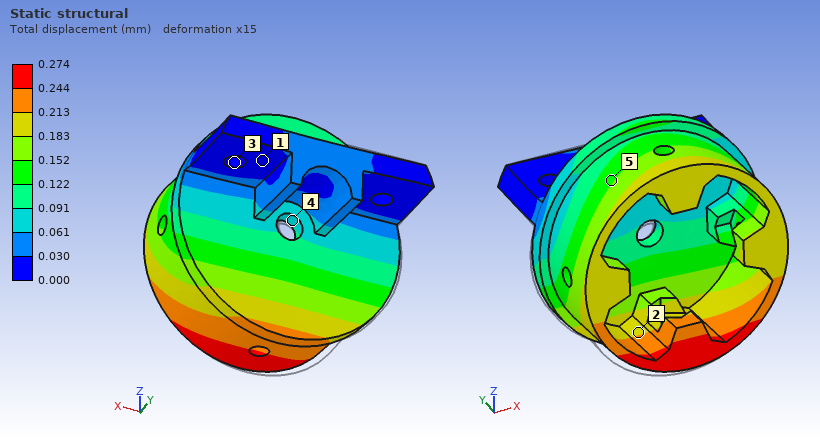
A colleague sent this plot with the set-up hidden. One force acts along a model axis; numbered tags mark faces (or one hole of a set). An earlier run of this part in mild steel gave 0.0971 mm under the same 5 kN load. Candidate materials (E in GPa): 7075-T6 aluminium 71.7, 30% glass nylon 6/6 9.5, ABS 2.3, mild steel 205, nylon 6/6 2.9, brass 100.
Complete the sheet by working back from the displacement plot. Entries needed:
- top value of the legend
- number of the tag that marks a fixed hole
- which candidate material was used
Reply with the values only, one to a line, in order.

0.274 mm
3
7075-T6 aluminium
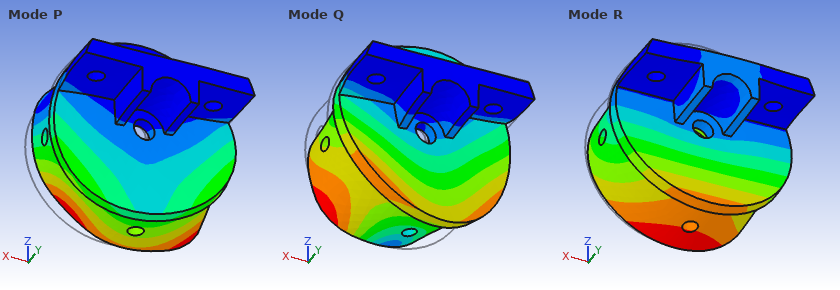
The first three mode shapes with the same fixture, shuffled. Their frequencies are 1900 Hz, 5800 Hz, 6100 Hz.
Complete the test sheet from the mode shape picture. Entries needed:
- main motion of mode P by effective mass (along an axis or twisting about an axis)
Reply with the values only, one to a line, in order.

along X
